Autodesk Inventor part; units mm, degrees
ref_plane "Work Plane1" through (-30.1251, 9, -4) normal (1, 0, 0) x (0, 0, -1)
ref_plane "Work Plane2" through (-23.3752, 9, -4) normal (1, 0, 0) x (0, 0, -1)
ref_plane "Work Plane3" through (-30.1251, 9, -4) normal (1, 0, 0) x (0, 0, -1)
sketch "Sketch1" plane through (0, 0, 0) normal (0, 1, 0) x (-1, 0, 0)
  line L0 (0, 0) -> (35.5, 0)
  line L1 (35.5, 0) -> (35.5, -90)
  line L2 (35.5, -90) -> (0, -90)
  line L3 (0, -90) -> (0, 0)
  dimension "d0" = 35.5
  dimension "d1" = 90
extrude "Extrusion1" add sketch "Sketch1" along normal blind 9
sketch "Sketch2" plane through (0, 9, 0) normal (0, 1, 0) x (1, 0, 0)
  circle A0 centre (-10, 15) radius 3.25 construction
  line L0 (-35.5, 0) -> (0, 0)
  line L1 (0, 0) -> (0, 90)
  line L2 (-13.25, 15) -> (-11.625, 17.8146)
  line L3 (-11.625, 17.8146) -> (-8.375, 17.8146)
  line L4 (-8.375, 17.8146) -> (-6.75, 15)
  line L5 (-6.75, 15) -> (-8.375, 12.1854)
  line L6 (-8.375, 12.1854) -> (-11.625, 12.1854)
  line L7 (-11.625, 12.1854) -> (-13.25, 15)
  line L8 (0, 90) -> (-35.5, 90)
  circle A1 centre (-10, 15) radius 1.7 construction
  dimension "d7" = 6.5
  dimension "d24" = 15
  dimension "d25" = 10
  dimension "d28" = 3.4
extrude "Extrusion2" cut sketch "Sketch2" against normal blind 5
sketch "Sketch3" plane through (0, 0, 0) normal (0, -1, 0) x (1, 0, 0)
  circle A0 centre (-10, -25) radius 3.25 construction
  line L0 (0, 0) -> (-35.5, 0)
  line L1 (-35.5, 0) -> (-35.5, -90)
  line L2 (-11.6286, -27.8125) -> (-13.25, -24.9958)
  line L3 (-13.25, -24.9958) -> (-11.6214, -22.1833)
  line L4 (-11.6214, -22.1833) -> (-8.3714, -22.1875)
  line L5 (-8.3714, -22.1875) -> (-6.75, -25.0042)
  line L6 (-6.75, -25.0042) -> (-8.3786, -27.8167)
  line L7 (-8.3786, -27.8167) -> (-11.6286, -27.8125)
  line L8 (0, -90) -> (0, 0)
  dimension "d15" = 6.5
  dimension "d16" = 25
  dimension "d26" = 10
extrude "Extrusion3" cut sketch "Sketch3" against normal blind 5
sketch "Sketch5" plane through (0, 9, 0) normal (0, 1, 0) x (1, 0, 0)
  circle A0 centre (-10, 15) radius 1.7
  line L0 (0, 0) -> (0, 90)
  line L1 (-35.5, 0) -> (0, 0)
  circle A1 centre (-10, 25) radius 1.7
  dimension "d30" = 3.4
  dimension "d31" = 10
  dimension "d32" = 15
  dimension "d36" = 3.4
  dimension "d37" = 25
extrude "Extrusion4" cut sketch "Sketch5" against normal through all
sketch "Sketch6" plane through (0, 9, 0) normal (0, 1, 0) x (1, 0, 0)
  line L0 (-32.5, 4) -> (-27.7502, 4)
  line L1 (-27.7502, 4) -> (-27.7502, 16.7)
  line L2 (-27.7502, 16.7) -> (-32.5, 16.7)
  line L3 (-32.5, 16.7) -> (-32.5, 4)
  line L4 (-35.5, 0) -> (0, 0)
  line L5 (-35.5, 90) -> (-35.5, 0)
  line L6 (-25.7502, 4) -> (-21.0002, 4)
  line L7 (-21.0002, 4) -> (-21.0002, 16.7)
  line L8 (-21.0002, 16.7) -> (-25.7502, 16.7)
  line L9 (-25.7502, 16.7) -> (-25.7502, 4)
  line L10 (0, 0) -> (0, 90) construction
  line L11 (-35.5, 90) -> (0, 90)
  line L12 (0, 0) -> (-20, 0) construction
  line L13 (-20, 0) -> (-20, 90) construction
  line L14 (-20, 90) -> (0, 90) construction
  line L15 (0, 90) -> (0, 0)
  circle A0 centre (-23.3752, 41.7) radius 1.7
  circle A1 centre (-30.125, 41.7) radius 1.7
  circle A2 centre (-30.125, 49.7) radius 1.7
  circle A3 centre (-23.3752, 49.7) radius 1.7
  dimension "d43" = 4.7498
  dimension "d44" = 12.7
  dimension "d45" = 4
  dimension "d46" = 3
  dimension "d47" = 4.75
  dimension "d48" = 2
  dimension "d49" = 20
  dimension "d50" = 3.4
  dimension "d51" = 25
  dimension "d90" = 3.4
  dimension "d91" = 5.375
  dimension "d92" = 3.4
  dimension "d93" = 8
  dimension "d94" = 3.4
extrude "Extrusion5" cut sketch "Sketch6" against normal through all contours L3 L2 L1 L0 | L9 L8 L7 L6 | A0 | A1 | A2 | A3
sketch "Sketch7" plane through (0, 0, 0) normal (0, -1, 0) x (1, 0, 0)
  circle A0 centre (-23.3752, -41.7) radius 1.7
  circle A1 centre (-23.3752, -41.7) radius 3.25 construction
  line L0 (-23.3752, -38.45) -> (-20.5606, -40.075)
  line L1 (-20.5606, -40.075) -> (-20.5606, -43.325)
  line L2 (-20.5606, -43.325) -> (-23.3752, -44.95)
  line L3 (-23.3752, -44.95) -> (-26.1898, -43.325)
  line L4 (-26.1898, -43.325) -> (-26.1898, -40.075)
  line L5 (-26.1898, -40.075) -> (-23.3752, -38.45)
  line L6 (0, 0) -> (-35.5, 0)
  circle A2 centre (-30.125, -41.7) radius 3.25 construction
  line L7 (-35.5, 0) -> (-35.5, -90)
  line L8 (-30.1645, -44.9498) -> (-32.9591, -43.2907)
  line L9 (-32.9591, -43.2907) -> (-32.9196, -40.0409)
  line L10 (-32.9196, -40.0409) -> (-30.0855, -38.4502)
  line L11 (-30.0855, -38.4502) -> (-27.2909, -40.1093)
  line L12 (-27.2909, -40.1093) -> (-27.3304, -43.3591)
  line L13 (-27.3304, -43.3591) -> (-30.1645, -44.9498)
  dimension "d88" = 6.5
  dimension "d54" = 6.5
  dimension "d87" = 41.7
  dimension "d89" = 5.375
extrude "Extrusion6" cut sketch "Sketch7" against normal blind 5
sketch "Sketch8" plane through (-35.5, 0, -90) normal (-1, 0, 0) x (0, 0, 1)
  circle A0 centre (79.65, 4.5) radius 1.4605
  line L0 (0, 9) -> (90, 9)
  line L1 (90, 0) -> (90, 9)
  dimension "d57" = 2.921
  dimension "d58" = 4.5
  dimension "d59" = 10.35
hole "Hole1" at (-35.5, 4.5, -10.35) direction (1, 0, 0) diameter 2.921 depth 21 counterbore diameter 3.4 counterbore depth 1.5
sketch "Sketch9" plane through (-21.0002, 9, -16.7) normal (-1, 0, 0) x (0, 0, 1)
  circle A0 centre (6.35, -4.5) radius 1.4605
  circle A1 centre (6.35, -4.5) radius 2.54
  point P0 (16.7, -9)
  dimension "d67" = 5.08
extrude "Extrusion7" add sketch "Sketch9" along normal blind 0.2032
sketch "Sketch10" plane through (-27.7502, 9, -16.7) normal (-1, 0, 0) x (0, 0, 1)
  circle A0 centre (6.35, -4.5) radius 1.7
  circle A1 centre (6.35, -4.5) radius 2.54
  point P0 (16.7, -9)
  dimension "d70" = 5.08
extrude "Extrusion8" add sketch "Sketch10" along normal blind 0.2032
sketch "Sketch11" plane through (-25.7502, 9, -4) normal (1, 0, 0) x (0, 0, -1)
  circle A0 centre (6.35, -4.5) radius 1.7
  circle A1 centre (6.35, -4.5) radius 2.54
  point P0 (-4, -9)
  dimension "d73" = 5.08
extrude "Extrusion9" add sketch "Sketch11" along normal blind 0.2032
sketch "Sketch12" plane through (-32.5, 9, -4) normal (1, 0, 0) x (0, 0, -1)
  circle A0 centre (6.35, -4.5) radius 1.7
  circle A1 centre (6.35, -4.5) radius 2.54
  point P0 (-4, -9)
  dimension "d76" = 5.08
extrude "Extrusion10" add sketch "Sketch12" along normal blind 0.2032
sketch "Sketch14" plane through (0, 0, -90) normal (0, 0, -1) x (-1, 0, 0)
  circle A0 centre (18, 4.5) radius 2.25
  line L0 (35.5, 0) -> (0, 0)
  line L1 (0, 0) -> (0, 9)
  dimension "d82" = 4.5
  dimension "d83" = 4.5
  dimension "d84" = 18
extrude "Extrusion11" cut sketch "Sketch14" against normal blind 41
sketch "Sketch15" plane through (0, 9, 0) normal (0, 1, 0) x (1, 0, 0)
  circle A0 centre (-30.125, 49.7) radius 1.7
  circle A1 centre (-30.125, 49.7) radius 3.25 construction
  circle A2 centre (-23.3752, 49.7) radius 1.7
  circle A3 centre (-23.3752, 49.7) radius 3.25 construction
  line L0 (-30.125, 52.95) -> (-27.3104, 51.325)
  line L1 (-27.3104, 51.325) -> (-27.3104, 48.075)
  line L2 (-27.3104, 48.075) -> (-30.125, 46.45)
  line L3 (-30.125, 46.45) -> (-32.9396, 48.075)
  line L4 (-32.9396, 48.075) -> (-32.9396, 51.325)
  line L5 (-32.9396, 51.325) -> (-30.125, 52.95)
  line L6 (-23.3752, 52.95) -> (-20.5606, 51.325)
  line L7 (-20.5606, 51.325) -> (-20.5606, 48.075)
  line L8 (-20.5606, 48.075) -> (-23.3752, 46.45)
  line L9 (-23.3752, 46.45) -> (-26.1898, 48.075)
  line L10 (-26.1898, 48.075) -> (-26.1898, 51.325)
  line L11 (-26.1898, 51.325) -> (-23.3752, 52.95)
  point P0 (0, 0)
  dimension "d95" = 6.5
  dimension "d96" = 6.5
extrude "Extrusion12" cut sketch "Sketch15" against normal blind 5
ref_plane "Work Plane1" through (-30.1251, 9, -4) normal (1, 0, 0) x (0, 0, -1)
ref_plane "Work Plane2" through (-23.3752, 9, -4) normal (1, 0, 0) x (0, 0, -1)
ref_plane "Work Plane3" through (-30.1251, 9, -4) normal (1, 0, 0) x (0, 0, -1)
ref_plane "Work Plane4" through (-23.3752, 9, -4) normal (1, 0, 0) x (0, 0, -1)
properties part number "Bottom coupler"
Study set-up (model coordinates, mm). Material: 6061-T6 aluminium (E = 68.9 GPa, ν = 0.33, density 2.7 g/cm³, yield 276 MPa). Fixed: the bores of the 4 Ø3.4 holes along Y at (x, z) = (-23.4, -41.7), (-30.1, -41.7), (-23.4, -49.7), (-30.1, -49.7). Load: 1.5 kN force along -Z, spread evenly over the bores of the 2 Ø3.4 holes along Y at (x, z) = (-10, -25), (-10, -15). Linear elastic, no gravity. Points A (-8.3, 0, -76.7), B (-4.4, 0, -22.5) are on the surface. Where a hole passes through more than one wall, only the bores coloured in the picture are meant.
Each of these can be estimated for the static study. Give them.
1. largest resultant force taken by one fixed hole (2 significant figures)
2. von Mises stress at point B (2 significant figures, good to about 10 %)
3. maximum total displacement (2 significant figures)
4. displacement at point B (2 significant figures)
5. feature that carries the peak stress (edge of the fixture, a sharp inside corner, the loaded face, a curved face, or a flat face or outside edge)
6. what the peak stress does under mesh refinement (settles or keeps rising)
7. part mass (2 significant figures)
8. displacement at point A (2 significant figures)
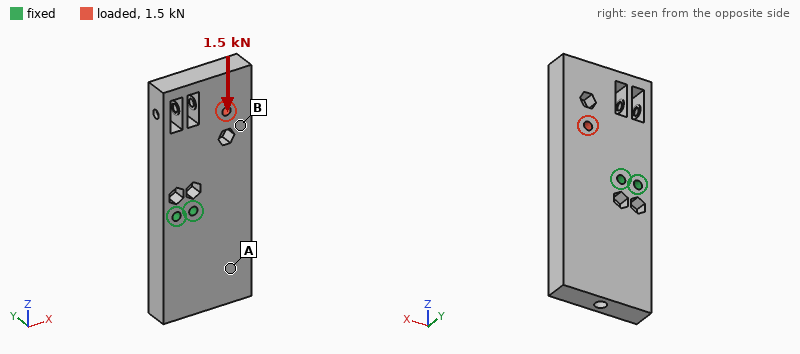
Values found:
1.5 kN
12 MPa
32 µm
21 µm
edge of the fixture
keeps rising
70 g
16 µm
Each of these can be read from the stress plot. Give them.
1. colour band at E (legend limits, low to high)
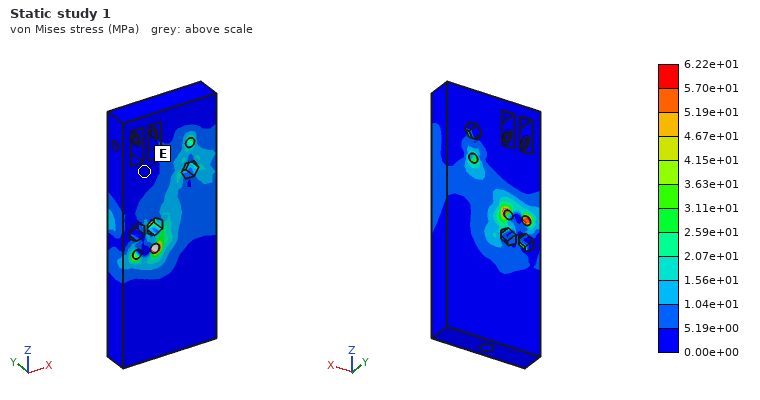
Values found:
0.00e+00 to 5.19e+00 MPa
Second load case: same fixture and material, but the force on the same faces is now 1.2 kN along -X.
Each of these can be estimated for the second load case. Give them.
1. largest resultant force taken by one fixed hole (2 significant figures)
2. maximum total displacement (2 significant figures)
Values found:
1.6 kN
43 µm
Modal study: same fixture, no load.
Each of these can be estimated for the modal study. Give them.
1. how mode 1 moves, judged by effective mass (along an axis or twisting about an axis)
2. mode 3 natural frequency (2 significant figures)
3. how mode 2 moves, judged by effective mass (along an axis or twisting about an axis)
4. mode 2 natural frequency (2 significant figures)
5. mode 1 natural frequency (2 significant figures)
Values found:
twisting about X
4500 Hz
along Y
3500 Hz
2800 Hz
